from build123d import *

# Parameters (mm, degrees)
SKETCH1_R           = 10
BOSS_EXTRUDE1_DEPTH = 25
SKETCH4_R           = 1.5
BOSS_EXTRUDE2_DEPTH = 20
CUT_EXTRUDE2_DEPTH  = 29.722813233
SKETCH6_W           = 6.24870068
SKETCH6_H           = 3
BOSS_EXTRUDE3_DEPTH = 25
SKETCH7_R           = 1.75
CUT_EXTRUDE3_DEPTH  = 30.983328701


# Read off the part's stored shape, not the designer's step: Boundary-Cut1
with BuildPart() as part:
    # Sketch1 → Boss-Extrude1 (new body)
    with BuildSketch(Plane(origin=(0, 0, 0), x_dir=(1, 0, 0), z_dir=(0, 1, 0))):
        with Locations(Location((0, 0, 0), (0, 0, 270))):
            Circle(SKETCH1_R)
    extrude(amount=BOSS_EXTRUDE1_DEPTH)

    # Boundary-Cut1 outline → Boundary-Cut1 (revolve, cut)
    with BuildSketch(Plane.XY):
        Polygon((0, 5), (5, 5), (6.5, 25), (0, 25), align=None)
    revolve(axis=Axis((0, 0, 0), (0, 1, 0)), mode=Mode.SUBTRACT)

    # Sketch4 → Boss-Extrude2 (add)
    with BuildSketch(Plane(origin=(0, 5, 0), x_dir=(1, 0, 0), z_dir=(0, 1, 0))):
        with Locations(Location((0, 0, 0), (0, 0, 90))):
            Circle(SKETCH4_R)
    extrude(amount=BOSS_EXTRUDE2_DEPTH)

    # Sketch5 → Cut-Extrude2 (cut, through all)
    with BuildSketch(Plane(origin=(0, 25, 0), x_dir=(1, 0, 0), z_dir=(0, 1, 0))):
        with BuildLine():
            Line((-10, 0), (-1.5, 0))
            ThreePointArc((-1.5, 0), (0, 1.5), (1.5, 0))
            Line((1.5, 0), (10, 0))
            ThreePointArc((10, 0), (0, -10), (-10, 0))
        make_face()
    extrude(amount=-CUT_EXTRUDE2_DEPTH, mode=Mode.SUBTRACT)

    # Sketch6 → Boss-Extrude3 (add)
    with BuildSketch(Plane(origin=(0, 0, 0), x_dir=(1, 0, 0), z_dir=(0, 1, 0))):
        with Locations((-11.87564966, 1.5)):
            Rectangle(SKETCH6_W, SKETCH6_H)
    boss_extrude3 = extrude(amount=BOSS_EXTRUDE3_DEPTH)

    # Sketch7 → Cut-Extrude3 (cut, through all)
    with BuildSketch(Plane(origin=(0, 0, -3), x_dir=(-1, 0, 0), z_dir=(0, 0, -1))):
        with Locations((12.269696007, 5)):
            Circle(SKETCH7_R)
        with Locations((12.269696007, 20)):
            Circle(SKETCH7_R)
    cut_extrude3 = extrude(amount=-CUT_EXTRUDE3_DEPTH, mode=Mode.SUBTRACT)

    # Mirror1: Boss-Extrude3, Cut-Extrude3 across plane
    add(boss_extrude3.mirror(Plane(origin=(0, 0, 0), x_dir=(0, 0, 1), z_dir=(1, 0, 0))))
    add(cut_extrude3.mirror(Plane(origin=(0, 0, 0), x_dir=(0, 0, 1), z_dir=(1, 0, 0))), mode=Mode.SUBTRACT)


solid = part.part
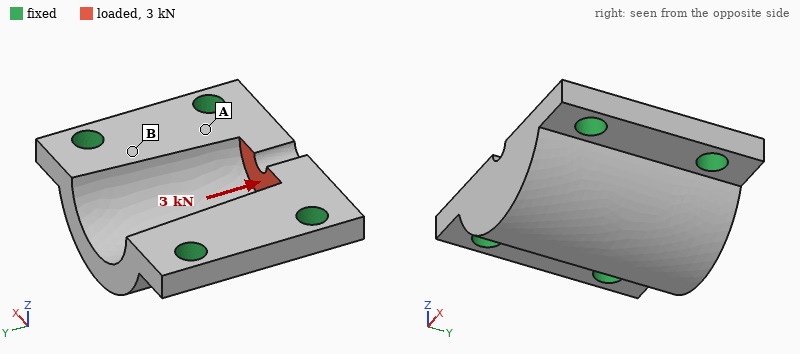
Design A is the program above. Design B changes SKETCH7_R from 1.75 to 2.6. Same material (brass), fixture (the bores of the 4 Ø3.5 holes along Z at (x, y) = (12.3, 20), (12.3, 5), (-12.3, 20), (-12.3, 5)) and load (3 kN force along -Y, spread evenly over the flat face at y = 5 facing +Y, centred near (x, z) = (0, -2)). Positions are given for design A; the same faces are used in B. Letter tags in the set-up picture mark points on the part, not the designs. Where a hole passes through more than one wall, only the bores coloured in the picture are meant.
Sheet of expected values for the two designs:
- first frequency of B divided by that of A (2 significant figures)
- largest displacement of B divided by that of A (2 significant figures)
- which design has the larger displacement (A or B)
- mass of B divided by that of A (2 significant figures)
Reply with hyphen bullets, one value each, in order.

- 1.2
- 0.91
- A
- 0.96
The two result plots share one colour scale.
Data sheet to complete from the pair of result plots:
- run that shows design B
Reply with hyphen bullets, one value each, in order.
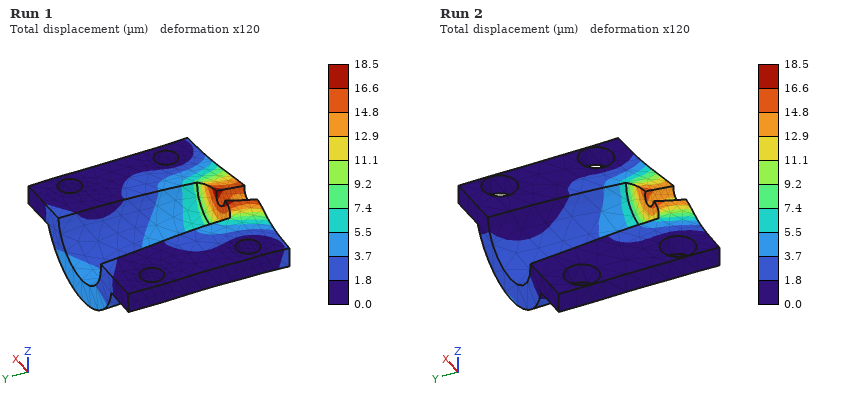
- Run 2
